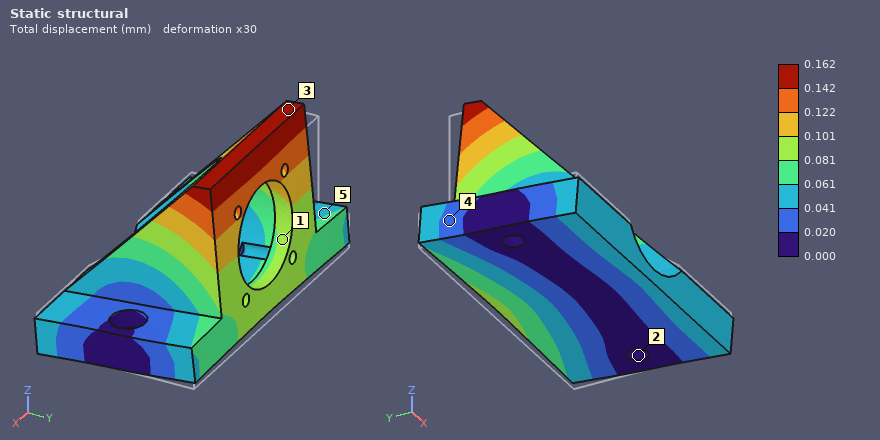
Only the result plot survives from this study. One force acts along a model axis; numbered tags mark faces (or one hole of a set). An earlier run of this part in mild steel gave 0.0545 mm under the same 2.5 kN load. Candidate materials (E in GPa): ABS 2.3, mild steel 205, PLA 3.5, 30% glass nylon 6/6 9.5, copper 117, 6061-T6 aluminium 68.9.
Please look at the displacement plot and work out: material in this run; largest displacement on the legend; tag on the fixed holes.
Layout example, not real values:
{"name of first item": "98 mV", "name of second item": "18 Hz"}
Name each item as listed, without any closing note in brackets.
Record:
{"material in this run": "6061-T6 aluminium", "largest displacement on the legend": "0.162 mm", "tag on the fixed holes": "2"}
